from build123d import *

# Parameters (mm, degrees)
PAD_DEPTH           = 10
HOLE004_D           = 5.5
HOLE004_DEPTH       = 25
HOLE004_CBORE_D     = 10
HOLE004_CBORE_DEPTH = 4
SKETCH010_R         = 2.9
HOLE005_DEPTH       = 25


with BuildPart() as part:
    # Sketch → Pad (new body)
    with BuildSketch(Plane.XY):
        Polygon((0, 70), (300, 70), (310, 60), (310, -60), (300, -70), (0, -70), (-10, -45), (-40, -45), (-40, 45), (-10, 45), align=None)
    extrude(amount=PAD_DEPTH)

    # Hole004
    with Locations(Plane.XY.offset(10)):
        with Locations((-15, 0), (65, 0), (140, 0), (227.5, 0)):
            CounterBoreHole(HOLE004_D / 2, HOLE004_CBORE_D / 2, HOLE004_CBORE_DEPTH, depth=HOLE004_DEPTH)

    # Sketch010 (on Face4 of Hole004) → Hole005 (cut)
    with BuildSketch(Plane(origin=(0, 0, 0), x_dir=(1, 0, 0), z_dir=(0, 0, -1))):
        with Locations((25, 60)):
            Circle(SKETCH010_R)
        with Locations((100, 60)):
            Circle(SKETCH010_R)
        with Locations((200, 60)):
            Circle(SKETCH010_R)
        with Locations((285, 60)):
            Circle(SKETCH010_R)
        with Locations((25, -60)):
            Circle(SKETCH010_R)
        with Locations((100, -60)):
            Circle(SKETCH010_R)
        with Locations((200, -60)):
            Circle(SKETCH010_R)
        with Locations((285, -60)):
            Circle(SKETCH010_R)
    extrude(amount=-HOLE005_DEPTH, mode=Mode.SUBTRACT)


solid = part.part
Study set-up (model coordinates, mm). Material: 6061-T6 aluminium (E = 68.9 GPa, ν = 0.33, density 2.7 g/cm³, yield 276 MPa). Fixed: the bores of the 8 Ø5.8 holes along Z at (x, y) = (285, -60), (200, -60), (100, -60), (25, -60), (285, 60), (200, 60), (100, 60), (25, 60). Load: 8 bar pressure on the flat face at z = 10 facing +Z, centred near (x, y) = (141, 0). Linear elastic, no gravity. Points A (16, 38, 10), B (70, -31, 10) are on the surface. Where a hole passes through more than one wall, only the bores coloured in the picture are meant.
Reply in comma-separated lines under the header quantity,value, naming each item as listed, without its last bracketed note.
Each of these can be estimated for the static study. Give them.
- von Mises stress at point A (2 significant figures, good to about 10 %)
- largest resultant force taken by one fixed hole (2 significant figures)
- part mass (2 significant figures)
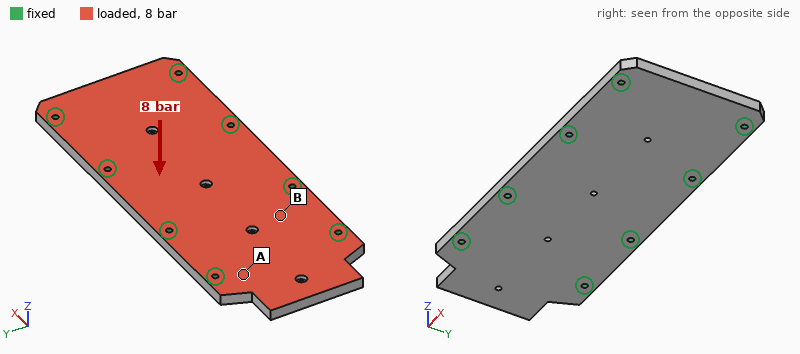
quantity,value
von Mises stress at point A,52 MPa
largest resultant force taken by one fixed hole,5.3 kN
part mass,1.3 kg
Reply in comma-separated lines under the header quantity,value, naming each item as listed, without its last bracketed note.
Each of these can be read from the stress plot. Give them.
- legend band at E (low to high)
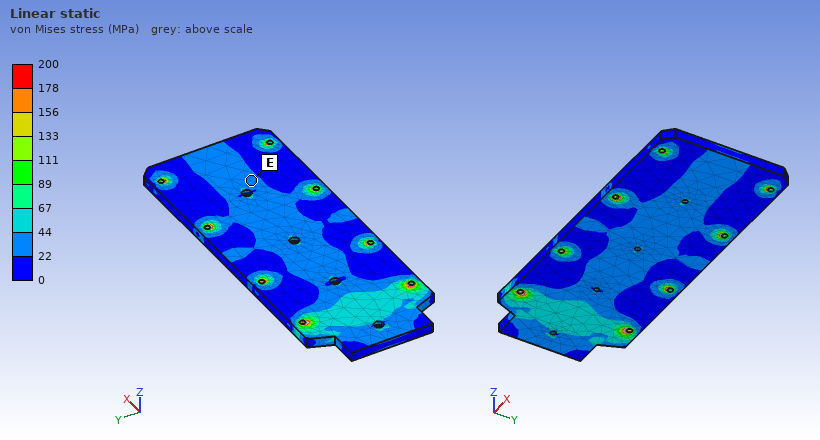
quantity,value
legend band at E,22 to 44 MPa
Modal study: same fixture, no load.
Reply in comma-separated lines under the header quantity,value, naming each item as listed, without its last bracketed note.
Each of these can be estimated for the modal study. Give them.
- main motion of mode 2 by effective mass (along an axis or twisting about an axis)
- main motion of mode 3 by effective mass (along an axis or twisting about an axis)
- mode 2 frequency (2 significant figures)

quantity,value
main motion of mode 2 by effective mass,along Z
main motion of mode 3 by effective mass,twisting about Y
mode 2 frequency,2500 Hz
